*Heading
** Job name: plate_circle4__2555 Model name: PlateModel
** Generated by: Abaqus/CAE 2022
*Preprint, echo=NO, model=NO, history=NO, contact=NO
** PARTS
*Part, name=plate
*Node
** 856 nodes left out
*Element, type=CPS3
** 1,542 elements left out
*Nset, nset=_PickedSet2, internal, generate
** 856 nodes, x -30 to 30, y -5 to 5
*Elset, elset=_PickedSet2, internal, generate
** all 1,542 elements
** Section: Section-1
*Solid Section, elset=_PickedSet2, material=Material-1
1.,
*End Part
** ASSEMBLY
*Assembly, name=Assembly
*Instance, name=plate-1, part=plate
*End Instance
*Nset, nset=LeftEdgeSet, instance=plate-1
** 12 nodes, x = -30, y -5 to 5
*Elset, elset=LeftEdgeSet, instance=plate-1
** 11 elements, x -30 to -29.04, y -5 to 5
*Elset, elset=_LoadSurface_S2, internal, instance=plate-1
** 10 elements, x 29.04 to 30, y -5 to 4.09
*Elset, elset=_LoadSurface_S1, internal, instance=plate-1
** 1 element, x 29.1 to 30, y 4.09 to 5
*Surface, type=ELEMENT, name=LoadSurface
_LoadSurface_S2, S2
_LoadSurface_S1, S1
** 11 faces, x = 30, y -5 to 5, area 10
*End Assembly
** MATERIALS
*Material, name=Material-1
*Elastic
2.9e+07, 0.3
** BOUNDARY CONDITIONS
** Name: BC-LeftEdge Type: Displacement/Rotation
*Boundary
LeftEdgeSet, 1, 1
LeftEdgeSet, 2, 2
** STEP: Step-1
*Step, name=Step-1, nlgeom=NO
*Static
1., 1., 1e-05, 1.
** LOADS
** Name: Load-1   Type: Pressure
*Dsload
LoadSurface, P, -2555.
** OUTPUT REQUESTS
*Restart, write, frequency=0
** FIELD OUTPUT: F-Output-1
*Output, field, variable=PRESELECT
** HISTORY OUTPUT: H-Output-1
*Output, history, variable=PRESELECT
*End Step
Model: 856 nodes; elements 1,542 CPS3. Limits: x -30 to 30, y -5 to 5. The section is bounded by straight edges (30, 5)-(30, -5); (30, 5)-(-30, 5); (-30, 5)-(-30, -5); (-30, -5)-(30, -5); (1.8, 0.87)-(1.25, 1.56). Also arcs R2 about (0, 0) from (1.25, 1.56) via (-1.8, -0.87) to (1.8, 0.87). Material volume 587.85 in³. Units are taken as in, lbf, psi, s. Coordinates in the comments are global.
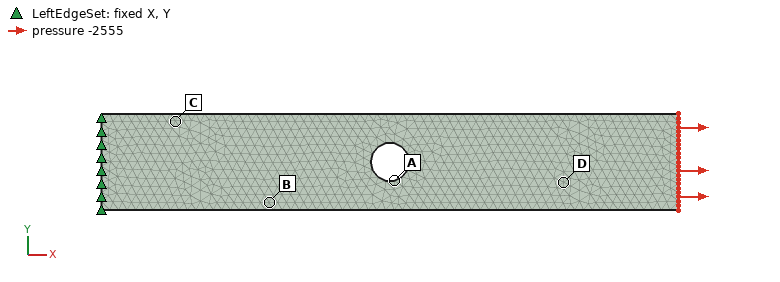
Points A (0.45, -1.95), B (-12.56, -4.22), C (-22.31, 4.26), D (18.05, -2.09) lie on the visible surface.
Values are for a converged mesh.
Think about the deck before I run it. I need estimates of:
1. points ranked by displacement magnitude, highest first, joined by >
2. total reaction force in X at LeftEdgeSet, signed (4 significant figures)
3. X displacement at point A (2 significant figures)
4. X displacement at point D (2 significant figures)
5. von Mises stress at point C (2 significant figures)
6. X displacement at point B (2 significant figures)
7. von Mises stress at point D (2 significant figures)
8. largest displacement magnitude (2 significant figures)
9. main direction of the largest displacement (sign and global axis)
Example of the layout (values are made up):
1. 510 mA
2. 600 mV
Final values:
1. D > A > B > C
2. -25550 lbf
3. 0.0030 in
4. 0.0046 in
5. 2500 psi
6. 0.0015 in
7. 2600 psi
8. 0.0057 in
9. +X
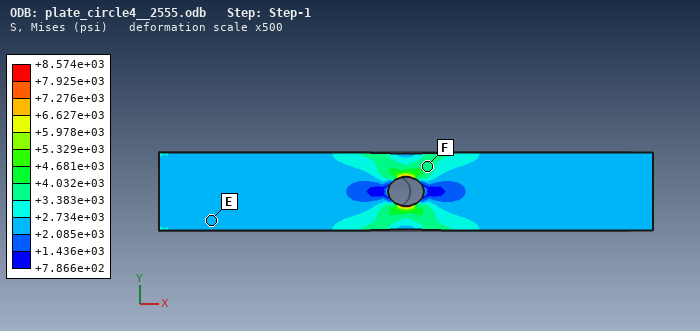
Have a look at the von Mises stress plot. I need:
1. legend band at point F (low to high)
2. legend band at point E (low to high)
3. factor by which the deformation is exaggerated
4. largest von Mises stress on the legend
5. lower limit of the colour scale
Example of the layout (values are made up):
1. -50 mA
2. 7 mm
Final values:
1. +3.383e+03 to +4.032e+03 psi
2. +2.085e+03 to +2.734e+03 psi
3. 500
4. +8.574e+03 psi
5. +7.866e+02 psi
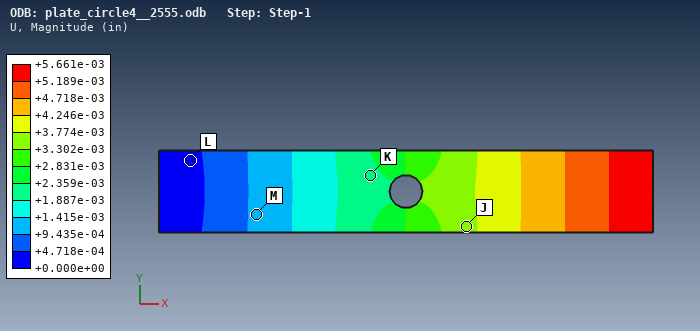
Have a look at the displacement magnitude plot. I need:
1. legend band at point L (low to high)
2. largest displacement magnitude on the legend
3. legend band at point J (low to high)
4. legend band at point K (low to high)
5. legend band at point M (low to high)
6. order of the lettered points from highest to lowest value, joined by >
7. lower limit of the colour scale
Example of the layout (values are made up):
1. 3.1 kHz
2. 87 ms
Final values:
1. +0.000e+00 to +4.718e-04 in
2. +5.661e-03 in
3. +3.302e-03 to +3.774e-03 in
4. +1.887e-03 to +2.359e-03 in
5. +9.435e-04 to +1.415e-03 in
6. J > K > M > L
7. +0.000e+00 in
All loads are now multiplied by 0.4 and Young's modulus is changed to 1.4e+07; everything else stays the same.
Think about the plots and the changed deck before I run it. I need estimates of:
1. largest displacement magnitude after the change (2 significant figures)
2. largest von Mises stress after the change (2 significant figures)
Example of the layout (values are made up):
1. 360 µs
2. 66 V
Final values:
1. 0.0047 in
2. 3400 psi
